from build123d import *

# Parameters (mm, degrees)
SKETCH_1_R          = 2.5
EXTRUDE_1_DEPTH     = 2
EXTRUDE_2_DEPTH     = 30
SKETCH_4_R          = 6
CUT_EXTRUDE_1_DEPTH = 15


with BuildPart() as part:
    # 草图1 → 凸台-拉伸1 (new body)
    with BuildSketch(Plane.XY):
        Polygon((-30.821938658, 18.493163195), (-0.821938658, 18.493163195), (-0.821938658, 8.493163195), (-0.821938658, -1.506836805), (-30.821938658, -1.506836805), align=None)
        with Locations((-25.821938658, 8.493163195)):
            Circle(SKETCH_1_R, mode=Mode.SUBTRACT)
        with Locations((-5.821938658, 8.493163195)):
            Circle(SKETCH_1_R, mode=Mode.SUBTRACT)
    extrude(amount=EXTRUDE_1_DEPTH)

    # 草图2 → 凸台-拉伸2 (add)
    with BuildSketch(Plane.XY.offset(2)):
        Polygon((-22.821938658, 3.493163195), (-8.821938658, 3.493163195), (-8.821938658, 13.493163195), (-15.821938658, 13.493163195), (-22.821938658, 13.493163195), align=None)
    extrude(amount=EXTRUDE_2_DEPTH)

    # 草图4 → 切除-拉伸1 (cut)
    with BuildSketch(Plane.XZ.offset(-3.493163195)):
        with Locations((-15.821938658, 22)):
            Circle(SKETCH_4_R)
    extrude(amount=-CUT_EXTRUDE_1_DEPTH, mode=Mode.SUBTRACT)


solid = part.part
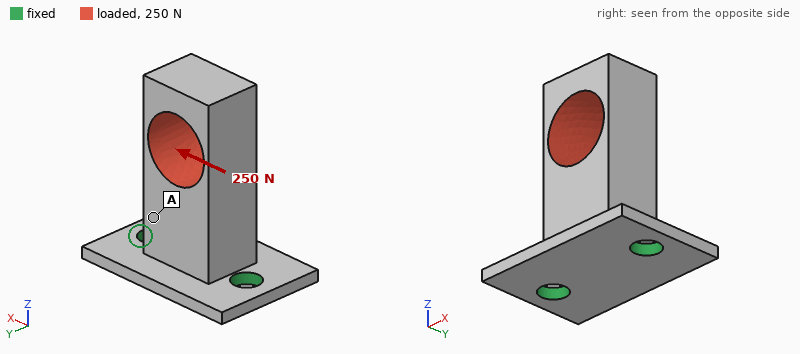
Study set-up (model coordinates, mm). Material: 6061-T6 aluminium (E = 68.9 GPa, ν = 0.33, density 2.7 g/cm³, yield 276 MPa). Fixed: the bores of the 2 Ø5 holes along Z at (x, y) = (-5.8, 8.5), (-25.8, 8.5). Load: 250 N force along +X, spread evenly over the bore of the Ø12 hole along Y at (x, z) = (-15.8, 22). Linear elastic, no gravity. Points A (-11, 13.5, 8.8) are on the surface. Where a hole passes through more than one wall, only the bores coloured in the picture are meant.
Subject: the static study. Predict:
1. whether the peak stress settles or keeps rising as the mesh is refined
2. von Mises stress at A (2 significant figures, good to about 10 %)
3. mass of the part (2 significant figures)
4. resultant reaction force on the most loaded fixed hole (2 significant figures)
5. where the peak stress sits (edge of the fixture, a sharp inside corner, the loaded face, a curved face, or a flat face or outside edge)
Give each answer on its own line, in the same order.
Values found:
keeps rising
6.8 MPa
11 g
370 N
a sharp inside corner
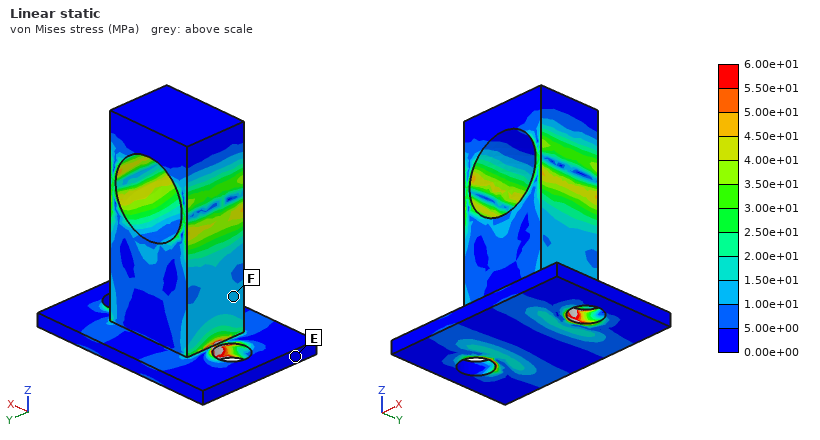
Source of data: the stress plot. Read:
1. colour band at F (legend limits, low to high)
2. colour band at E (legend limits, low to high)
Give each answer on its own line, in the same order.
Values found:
1.00e+01 to 1.50e+01 MPa
0.00e+00 to 5.00e+00 MPa
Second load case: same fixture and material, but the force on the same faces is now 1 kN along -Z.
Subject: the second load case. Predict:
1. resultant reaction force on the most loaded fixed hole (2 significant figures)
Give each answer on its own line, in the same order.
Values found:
540 N
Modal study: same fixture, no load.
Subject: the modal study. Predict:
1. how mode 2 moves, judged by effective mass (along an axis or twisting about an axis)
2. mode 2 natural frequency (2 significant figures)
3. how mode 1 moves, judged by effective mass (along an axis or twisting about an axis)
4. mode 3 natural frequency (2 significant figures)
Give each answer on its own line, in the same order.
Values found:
along X
6700 Hz
along Y
17 kHz
